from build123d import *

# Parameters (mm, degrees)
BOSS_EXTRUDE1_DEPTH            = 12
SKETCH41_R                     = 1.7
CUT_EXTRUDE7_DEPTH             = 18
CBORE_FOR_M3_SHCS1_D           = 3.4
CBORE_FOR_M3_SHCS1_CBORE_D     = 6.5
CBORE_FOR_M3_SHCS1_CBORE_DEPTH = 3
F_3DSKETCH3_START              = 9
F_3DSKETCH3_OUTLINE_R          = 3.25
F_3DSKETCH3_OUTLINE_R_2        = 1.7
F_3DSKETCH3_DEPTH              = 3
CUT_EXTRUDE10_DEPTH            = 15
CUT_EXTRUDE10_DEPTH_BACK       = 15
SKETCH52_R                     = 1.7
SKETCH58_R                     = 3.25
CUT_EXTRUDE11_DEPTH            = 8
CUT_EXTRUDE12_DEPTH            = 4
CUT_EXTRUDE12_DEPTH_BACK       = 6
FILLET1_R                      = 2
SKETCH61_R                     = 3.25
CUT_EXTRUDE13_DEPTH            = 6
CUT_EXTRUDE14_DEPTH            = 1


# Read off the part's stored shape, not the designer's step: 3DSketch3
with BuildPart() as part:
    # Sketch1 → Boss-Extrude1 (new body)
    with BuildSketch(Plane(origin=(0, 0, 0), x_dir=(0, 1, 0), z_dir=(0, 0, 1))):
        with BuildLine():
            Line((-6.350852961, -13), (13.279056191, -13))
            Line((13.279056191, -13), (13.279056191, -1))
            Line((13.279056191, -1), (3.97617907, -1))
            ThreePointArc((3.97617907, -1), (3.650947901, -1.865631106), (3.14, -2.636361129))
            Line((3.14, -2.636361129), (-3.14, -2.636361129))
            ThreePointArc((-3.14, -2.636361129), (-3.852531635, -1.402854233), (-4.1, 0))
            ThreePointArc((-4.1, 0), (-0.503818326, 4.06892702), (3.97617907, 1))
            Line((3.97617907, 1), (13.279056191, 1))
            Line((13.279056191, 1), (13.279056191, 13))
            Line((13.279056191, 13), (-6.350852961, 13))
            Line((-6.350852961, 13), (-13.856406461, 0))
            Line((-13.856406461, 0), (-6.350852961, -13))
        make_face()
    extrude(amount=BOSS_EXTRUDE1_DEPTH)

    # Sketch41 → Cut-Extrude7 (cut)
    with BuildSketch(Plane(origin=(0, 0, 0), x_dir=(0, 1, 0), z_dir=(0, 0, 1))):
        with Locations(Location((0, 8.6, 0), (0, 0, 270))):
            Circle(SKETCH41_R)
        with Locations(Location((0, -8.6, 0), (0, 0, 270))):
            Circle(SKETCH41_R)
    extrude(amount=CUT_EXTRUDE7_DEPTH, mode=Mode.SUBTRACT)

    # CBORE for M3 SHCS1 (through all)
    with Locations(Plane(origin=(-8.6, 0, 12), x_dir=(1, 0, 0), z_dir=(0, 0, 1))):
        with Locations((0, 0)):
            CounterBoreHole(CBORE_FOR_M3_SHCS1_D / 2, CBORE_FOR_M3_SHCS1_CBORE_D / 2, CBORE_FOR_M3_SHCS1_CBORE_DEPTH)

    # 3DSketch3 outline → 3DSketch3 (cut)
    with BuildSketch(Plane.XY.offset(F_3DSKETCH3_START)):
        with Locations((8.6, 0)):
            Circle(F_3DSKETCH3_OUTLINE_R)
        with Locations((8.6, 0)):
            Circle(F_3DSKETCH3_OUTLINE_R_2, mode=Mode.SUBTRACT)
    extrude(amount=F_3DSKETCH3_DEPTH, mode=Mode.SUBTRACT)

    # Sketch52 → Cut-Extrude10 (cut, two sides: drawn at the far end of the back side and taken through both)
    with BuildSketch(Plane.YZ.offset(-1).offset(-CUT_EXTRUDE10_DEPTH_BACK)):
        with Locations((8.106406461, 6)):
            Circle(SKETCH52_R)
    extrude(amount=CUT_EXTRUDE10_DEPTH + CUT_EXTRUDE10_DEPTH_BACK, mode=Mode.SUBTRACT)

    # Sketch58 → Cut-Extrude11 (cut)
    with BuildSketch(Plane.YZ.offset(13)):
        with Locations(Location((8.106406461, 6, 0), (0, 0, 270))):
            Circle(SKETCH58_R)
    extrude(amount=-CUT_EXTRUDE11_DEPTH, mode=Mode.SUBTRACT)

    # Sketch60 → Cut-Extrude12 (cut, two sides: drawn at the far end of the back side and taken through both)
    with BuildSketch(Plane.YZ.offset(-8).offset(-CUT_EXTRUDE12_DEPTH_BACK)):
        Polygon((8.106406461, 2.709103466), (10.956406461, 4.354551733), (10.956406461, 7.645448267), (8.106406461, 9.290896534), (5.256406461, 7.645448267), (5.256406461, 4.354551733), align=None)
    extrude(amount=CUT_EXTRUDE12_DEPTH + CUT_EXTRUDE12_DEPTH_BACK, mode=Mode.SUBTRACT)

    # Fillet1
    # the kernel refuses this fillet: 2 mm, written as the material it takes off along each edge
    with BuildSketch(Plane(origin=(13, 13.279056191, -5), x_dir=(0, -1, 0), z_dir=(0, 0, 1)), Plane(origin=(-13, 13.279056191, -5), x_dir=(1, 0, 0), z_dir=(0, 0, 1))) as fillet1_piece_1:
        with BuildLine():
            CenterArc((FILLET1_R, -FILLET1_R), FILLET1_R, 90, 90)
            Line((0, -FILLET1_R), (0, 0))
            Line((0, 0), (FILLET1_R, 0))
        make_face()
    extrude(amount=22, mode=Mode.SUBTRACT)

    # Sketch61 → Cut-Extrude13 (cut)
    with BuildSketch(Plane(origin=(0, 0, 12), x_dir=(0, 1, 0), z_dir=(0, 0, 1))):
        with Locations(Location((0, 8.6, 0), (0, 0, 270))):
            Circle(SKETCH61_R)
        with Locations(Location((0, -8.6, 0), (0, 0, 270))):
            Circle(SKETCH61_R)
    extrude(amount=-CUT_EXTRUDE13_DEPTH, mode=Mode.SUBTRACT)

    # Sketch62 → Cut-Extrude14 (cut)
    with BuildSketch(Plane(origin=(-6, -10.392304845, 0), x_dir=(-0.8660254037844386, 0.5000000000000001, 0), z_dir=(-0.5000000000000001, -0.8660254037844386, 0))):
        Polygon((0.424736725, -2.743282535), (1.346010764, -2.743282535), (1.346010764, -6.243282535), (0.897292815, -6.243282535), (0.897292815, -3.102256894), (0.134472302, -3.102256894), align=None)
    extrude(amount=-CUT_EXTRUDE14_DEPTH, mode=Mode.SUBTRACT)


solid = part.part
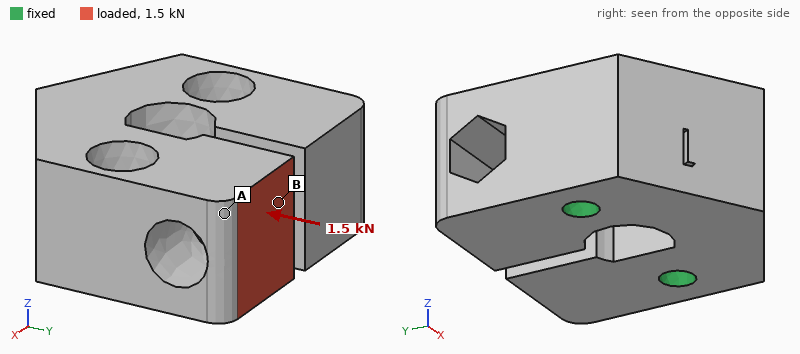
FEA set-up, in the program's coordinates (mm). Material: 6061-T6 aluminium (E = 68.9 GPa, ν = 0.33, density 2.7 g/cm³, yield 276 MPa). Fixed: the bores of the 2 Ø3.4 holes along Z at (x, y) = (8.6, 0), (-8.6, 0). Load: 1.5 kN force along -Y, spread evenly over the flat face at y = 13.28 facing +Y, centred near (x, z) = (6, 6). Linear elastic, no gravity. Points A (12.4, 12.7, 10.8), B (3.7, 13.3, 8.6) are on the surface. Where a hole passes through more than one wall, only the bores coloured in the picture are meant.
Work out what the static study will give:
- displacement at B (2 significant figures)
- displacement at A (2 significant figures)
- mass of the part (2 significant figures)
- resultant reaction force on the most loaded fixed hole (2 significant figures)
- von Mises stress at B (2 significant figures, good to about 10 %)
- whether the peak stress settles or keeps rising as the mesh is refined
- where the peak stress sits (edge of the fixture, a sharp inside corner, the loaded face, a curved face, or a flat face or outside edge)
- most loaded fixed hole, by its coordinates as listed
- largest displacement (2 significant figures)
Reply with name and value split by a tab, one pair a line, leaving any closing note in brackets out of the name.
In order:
displacement at B	13 µm
displacement at A	11 µm
mass of the part	15 g
resultant reaction force on the most loaded fixed hole	1.3 kN
von Mises stress at B	13 MPa
whether the peak stress settles or keeps rising as the mesh is refined	keeps rising
where the peak stress sits	edge of the fixture
most loaded fixed hole, by its coordinates as listed	(8.6, 0)
largest displacement	15 µm
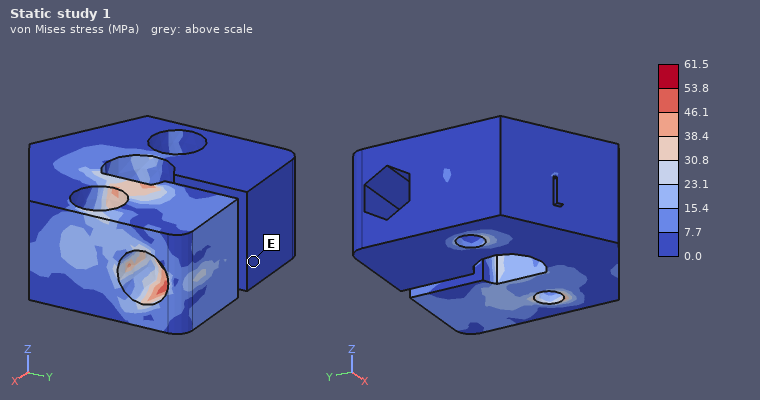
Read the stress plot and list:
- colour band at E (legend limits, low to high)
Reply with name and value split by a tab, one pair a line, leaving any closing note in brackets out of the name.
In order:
colour band at E	0.0 to 7.7 MPa
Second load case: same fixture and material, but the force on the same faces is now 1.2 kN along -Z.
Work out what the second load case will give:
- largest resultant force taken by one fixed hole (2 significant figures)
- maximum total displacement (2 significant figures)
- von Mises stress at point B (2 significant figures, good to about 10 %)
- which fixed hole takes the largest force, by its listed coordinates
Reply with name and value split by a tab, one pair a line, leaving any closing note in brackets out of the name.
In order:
largest resultant force taken by one fixed hole	1.3 kN
maximum total displacement	55 µm
von Mises stress at point B	33 MPa
which fixed hole takes the largest force, by its listed coordinates	(8.6, 0)
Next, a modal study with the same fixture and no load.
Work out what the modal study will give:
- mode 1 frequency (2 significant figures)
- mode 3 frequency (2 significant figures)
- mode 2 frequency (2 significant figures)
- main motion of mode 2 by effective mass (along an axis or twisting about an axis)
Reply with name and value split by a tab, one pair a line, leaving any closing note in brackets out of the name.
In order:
mode 1 frequency	17 kHz
mode 3 frequency	21 kHz
mode 2 frequency	19 kHz
main motion of mode 2 by effective mass	along X
